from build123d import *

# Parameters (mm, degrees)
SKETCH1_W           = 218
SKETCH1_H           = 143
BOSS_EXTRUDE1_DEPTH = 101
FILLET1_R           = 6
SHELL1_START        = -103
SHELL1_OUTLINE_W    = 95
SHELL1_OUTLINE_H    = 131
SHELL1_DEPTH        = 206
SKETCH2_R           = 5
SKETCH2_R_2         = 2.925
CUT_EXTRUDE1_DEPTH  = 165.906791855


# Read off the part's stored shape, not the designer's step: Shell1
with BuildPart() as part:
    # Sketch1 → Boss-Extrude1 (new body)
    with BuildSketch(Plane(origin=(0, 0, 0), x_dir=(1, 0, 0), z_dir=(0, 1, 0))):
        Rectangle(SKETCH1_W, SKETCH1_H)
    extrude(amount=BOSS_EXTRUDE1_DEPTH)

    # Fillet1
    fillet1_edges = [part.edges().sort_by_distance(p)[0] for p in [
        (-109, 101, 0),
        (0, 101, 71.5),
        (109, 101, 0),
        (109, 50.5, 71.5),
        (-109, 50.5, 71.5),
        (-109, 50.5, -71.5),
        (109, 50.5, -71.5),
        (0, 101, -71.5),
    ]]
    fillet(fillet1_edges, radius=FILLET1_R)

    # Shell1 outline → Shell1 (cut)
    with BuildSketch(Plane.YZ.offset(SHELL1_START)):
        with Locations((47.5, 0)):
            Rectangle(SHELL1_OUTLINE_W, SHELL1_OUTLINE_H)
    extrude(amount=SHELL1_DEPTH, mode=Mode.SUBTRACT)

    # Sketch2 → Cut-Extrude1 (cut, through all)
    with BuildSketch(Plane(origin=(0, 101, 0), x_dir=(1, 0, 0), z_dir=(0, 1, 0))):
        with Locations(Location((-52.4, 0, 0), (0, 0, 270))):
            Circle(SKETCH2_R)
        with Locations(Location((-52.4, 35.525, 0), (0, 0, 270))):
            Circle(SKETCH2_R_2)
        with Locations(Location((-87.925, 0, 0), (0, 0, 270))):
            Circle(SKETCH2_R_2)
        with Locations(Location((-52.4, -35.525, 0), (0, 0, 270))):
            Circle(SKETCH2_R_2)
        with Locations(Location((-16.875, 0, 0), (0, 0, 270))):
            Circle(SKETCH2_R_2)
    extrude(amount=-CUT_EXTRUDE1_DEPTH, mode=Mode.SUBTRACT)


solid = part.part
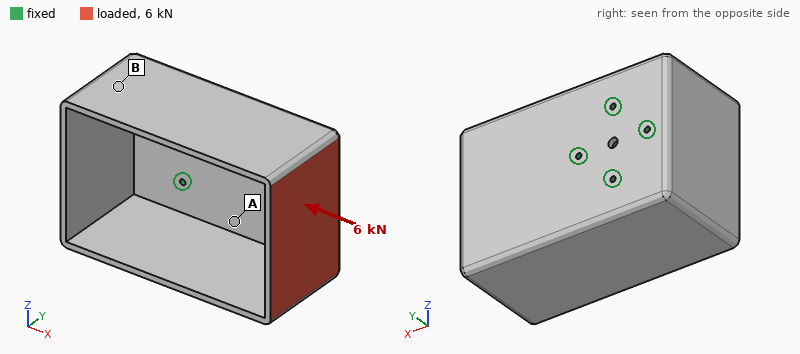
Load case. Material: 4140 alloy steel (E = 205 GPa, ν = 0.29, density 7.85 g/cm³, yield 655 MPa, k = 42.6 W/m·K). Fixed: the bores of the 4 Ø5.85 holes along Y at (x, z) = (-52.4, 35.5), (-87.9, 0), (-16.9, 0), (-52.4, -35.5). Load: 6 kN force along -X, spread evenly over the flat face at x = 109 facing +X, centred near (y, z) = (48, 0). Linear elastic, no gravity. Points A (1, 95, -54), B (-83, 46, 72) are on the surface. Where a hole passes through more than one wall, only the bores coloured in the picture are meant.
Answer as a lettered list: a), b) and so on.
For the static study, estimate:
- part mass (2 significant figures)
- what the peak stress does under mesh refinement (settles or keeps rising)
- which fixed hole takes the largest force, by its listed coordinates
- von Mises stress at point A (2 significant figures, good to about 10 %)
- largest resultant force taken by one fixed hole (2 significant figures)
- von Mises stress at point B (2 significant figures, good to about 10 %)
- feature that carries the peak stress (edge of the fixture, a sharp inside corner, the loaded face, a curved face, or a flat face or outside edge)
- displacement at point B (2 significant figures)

a) 4.5 kg
b) keeps rising
c) (-87.9, 0)
d) 17 MPa
e) 4.5 kN
f) 7.5 MPa
g) edge of the fixture
h) 0.089 mm
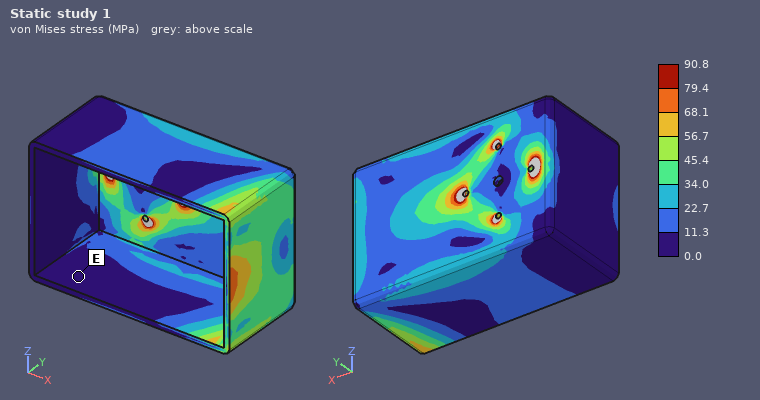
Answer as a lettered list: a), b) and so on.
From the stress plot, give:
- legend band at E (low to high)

a) 0.0 to 11.3 MPa
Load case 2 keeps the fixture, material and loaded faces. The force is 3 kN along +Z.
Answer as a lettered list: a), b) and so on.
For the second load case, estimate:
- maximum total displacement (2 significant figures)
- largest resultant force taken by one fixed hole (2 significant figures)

a) 0.53 mm
b) 4.4 kN
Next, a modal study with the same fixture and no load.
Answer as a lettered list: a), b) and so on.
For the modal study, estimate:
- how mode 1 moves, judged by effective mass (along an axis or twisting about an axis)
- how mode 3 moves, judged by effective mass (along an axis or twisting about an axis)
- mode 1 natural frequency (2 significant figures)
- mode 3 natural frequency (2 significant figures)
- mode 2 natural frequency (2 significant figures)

a) along Y
b) along Z
c) 270 Hz
d) 580 Hz
e) 310 Hz
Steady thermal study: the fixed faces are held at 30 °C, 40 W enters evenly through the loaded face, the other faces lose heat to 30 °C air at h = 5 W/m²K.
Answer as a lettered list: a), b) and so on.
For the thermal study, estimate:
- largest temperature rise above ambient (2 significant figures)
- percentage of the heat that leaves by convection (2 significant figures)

a) 75 K
b) 55 %
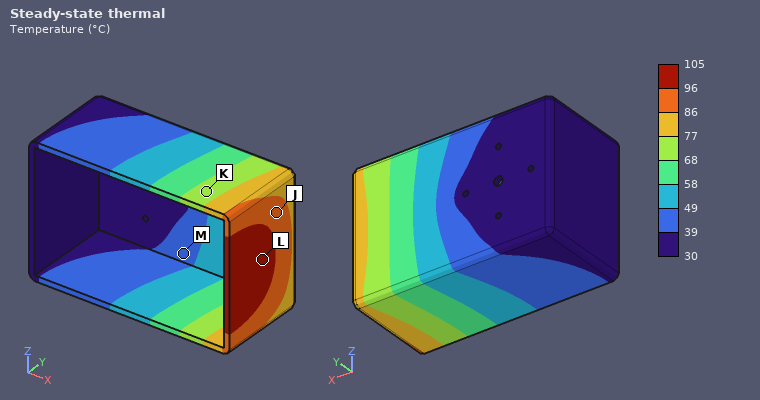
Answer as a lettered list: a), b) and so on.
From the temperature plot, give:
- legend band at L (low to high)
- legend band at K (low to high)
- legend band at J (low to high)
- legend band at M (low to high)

a) 96 to 105 °C
b) 68 to 77 °C
c) 86 to 96 °C
d) 39 to 49 °C
